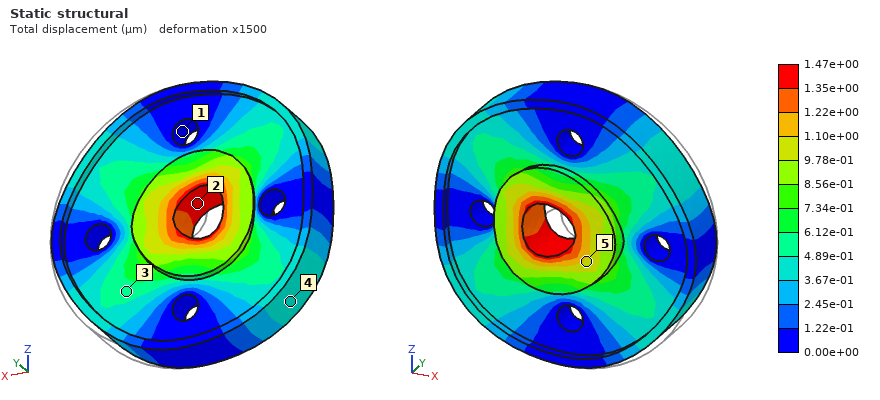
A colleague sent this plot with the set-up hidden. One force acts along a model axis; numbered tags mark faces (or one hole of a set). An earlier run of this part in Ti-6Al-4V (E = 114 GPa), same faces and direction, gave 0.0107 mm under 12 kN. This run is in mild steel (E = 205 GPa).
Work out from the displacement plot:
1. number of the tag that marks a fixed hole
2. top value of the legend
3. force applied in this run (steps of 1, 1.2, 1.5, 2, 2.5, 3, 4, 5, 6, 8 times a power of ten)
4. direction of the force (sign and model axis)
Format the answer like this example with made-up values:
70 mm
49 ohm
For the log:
1
1.47e+00 µm
3 kN
-X
